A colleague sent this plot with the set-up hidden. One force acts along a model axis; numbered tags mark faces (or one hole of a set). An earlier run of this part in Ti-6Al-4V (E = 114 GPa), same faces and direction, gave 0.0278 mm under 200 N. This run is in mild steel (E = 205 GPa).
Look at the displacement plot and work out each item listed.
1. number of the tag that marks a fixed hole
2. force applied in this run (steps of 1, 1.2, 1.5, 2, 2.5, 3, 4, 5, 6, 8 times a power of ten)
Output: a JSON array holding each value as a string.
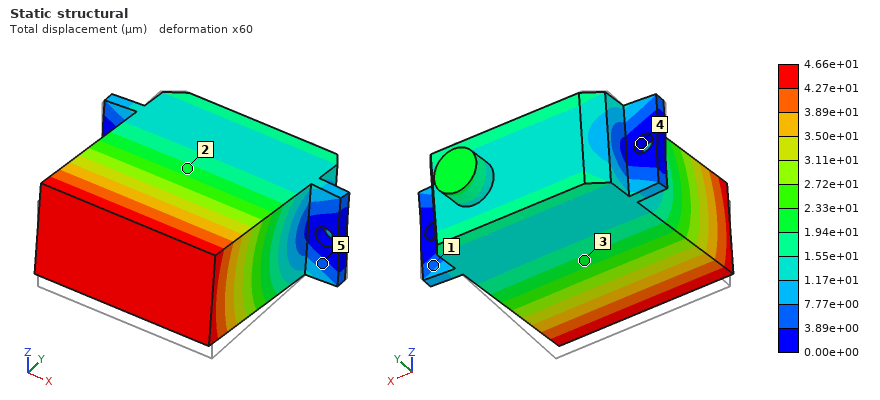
["4", "600 N"]
